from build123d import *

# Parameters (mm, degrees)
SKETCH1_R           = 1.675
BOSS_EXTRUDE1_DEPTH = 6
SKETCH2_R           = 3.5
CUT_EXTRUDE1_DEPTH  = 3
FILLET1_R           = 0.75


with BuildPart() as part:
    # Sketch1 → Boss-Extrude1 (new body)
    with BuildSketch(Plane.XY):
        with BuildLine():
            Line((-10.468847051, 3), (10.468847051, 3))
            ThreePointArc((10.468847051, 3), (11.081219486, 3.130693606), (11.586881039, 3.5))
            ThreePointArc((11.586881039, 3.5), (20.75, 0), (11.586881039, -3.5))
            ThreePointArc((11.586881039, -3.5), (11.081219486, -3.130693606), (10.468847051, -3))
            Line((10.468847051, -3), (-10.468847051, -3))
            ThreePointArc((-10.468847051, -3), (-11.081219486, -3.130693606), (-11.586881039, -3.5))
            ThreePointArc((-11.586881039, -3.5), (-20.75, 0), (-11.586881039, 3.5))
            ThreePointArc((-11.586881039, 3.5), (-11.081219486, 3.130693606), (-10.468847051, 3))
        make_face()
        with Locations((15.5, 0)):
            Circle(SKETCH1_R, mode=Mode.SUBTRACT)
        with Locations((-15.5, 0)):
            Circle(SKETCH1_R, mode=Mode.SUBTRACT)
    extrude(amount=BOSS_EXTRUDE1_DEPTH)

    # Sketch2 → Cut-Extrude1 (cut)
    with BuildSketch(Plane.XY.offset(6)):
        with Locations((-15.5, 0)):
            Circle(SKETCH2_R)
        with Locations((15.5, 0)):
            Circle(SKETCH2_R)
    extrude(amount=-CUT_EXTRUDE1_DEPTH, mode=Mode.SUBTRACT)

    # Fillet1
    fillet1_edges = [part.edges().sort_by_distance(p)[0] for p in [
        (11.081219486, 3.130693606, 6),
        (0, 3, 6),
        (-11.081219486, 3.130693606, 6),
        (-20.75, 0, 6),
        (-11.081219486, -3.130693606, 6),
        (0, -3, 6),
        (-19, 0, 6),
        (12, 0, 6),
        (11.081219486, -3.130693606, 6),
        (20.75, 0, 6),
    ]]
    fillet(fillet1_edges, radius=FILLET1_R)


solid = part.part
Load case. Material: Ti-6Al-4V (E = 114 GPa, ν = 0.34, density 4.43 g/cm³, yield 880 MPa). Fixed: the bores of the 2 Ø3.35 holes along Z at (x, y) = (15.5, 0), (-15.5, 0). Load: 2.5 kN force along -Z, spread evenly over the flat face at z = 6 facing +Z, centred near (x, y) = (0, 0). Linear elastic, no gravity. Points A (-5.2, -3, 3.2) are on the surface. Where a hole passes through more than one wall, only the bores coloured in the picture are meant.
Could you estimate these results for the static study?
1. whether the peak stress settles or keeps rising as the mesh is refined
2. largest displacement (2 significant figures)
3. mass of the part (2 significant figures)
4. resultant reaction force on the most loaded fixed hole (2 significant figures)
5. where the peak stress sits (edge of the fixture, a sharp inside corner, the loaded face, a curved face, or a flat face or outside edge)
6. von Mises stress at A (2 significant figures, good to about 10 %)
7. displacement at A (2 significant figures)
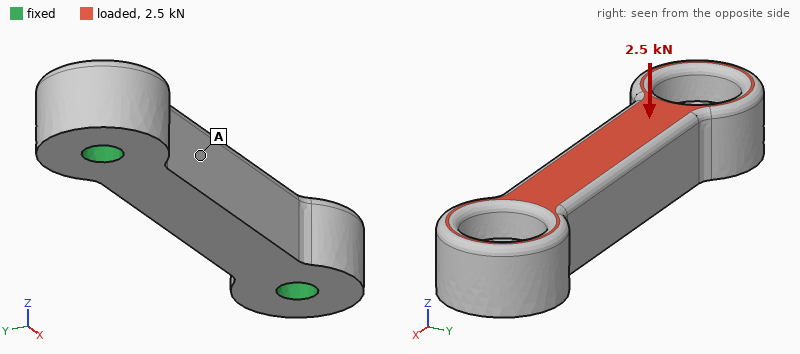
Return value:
keeps rising
33 µm
6.6 g
1.5 kN
edge of the fixture
50 MPa
27 µm
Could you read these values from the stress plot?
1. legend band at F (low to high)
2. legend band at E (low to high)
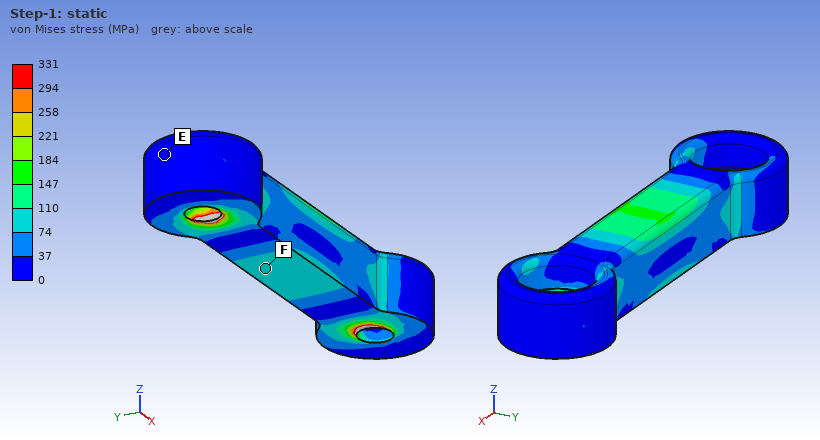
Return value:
74 to 110 MPa
0 to 37 MPa
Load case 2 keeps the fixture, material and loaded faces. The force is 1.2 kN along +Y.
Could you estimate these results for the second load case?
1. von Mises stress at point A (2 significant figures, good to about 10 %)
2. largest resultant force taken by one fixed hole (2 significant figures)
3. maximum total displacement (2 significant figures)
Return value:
45 MPa
600 N
24 µm
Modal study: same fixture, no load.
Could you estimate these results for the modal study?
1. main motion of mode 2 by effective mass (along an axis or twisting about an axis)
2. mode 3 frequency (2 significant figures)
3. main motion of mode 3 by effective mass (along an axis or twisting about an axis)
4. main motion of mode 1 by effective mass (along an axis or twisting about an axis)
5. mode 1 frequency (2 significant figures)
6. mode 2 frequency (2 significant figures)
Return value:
along Y
43 kHz
twisting about X
along Z
24 kHz
25 kHz
